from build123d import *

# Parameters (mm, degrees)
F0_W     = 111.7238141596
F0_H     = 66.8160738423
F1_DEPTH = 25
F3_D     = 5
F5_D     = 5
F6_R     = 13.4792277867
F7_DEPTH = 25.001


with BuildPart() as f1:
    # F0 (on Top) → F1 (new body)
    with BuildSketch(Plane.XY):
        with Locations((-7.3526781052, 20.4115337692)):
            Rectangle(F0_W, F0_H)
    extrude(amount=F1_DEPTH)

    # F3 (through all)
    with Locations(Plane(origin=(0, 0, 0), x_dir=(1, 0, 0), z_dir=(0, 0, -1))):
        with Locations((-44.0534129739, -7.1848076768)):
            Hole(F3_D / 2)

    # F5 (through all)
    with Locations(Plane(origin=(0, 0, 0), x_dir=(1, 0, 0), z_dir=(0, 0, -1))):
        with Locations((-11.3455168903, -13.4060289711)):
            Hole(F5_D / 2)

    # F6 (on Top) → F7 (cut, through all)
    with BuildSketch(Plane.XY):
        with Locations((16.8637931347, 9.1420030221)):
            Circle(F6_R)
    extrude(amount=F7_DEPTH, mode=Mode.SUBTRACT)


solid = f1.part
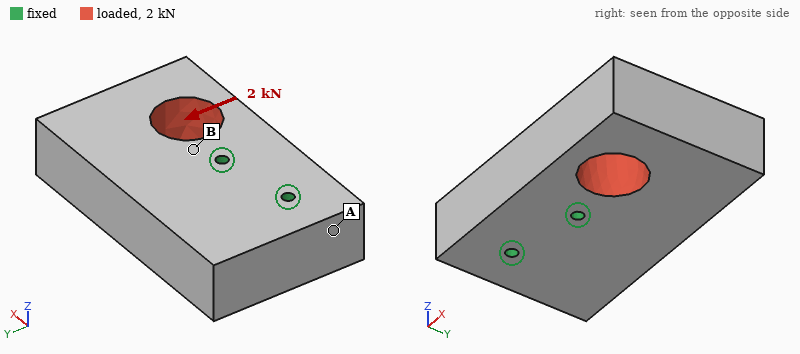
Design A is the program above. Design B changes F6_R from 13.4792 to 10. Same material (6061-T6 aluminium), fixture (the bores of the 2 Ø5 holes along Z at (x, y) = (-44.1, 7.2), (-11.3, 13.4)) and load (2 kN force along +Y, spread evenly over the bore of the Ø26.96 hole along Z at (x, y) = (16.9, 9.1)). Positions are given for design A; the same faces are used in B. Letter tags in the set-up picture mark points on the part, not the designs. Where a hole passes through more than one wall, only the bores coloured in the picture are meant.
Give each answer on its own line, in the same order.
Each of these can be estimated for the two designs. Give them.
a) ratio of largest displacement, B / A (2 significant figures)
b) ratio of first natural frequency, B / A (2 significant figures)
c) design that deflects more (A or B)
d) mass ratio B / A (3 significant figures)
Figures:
0.88
1.0
A
1.04
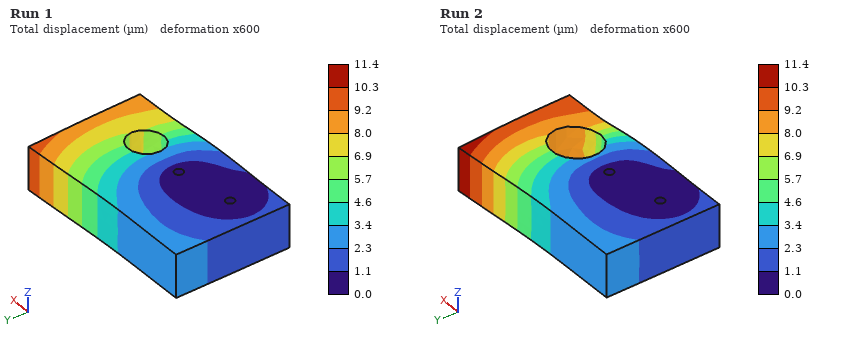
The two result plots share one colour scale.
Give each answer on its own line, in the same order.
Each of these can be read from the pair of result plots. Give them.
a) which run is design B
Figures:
Run 1
